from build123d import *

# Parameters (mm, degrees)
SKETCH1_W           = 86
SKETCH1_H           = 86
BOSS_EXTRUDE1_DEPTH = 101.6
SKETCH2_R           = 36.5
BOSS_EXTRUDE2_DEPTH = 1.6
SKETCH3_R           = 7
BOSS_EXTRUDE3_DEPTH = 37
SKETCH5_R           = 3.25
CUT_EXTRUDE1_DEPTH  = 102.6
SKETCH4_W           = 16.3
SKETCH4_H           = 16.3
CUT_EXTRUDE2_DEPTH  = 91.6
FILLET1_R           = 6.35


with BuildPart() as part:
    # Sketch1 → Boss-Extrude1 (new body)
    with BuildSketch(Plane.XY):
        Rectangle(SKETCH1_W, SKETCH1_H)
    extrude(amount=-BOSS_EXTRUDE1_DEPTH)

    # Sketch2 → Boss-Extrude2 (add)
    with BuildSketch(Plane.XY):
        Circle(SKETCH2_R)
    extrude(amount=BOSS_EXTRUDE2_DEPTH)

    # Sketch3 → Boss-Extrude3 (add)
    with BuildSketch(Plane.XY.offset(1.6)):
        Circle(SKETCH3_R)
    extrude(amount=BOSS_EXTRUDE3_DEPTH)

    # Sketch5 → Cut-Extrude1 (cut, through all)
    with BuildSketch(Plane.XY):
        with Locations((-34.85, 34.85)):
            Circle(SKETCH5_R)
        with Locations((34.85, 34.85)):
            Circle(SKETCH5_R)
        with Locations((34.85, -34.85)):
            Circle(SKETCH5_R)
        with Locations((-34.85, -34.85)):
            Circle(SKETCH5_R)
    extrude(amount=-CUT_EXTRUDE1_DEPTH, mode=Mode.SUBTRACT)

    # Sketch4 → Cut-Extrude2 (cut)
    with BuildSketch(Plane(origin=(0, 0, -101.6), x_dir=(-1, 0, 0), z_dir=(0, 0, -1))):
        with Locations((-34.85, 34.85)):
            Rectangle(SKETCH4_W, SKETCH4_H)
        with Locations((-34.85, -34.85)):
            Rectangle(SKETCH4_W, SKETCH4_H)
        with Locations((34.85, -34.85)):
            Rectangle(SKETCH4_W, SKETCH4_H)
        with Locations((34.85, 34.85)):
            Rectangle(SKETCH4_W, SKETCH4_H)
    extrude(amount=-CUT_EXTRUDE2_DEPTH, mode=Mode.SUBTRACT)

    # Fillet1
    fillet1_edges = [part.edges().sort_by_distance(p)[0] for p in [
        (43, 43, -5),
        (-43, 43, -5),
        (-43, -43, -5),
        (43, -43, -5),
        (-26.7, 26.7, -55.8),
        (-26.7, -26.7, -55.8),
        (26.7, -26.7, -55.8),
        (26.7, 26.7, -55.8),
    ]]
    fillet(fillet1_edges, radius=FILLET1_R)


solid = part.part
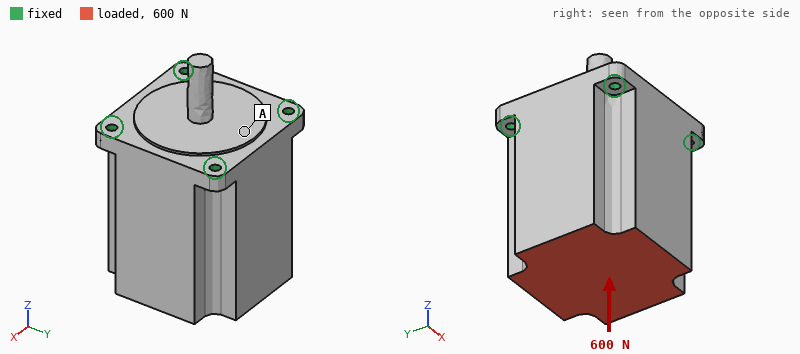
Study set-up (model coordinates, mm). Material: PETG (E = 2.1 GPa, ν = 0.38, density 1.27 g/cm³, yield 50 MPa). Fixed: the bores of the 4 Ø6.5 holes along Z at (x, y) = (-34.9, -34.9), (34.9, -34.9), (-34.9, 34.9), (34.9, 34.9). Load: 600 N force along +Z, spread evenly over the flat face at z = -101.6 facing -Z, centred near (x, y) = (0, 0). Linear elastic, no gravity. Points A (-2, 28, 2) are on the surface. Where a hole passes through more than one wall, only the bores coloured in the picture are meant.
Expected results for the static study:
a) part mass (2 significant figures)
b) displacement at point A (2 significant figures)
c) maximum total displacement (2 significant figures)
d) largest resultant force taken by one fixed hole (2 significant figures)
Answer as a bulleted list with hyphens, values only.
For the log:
- 850 g
- 13 µm
- 16 µm
- 160 N
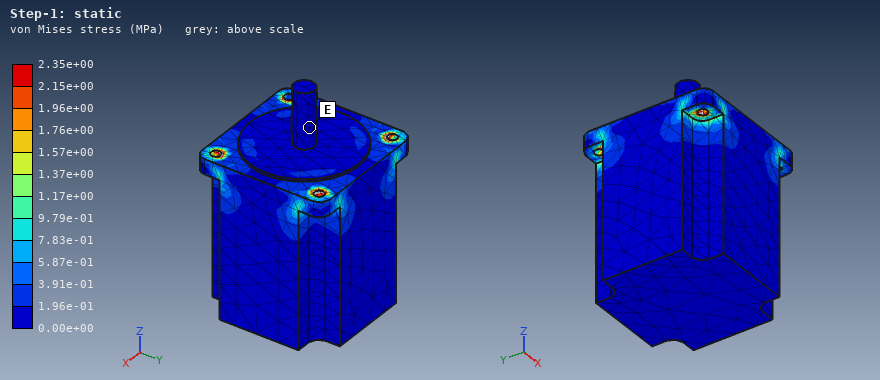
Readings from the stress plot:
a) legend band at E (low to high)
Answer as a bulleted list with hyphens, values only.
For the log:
- 0.00e+00 to 1.96e-01 MPa
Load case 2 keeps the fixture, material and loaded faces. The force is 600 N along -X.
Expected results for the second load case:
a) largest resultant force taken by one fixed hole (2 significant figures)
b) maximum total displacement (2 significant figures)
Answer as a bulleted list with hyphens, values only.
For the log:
- 480 N
- 0.15 mm
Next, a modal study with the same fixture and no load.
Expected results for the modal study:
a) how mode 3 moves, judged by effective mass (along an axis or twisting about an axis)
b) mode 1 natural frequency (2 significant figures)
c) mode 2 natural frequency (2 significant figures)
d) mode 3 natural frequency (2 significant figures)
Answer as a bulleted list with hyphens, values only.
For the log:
- along Z
- 620 Hz
- 620 Hz
- 1200 Hz
